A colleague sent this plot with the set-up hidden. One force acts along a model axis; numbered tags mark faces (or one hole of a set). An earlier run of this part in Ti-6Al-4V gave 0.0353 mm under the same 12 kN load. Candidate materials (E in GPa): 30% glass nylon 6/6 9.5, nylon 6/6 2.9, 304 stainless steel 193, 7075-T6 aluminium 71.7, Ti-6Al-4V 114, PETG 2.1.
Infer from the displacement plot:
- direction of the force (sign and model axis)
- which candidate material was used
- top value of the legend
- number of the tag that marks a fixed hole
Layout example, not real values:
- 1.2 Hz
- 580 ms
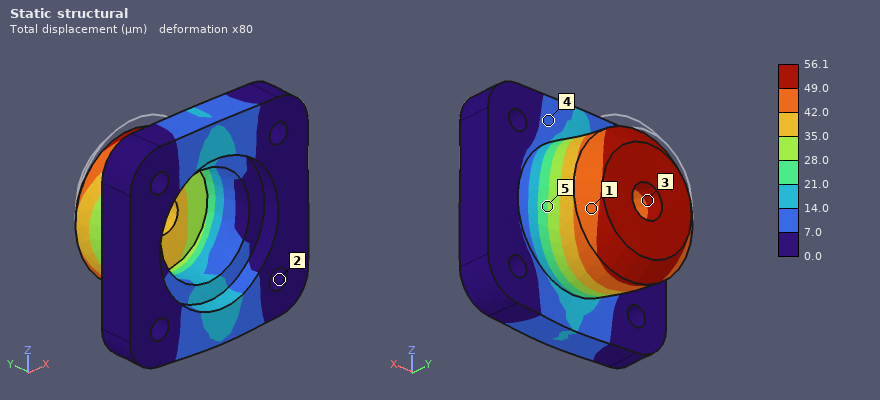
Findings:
- -Z
- 7075-T6 aluminium
- 56.1 µm
- 2
